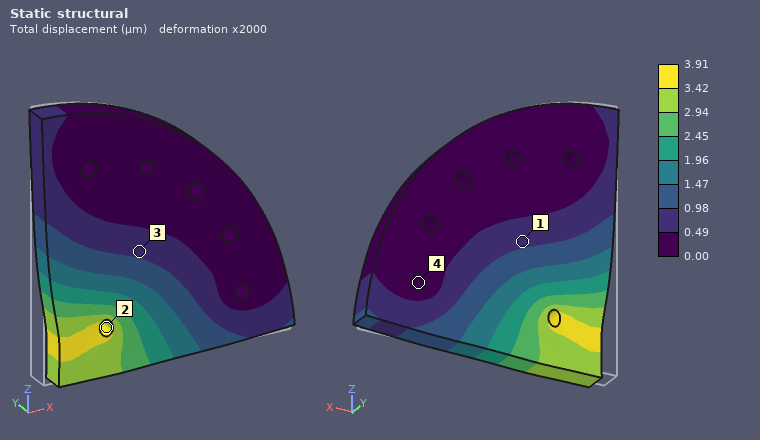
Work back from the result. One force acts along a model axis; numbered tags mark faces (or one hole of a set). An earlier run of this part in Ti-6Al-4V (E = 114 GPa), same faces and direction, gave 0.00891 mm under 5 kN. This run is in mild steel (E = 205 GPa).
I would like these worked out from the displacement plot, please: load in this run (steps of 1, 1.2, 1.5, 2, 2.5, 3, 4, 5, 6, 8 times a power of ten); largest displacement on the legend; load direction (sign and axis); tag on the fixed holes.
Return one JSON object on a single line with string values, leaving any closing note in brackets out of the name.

{"load in this run": "4 kN", "largest displacement on the legend": "3.91 µm", "load direction": "+X", "tag on the fixed holes": "4"}
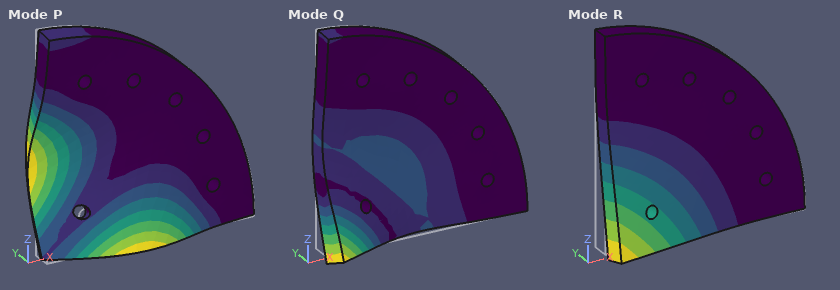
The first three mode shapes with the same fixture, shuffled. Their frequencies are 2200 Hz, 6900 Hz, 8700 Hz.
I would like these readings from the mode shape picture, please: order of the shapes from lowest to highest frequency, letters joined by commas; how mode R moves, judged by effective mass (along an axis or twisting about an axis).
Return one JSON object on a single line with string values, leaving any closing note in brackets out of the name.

{"order of the shapes from lowest to highest frequency, letters joined by commas": "R, P, Q", "how mode R moves, judged by effective mass": "along Y"}
